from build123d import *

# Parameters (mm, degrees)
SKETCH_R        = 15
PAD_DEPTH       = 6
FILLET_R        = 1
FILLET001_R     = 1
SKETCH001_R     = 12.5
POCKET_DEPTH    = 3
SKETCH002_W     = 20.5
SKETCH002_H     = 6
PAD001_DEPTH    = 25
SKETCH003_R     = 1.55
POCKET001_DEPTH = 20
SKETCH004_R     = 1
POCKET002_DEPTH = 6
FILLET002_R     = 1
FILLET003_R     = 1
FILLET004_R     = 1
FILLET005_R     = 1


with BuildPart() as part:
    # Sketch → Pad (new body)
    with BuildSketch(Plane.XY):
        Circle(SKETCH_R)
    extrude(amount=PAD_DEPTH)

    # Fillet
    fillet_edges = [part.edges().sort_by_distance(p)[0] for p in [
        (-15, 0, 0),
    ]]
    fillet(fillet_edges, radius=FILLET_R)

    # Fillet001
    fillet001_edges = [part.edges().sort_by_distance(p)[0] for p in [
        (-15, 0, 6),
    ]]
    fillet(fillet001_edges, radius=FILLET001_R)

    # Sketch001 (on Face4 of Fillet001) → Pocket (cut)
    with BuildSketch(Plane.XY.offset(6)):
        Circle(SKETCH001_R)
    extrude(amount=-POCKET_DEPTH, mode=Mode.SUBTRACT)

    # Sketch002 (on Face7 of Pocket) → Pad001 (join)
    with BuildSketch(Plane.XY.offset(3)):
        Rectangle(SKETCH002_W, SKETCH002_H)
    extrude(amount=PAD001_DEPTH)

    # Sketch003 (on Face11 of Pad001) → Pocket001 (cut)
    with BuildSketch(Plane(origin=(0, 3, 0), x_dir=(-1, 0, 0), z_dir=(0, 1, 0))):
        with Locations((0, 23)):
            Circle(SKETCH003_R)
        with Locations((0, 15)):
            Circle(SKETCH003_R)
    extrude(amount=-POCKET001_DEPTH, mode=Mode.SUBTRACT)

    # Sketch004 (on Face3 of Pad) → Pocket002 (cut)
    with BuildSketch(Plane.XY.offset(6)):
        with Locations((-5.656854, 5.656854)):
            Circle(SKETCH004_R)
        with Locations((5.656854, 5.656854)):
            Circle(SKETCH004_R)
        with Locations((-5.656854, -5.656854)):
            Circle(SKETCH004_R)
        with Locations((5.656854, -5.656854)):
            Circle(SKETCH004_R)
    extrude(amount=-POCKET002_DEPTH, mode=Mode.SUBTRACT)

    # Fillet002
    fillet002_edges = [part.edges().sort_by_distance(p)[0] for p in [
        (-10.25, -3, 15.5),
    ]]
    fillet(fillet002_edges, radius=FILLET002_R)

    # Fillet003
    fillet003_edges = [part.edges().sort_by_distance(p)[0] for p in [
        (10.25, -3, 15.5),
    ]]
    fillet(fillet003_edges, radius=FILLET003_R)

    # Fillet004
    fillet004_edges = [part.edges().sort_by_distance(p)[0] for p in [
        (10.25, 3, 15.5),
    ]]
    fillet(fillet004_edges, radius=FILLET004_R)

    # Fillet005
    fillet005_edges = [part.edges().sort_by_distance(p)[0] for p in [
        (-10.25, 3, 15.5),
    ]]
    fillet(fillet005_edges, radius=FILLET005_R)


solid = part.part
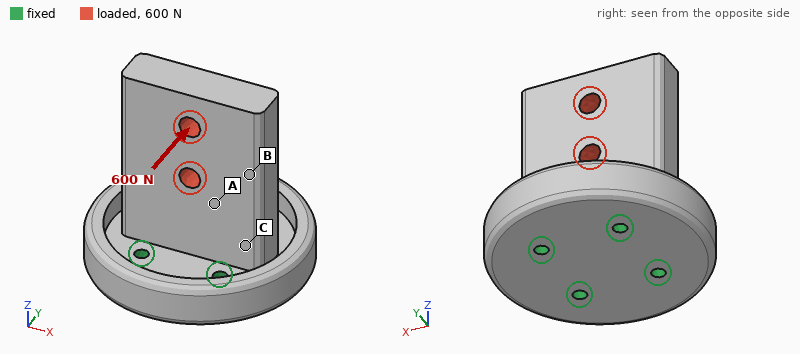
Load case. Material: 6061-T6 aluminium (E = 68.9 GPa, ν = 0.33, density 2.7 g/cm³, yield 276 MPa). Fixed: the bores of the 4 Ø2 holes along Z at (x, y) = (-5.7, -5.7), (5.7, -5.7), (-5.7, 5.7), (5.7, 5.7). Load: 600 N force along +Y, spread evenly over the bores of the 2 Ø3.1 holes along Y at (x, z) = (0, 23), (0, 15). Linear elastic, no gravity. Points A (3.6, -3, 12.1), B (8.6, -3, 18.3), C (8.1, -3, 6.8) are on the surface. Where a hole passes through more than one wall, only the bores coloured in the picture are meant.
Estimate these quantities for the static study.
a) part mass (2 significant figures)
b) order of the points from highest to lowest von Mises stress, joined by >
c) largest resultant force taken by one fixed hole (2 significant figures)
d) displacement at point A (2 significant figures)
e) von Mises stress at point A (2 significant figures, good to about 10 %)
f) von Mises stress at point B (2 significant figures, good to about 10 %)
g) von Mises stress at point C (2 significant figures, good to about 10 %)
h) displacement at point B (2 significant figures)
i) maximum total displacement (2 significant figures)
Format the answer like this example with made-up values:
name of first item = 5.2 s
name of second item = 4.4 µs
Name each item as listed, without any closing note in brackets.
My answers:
part mass = 15 g
order of the points from highest to lowest von Mises stress, joined by > = C > A > B
largest resultant force taken by one fixed hole = 550 N
displacement at point A = 29 µm
von Mises stress at point A = 37 MPa
von Mises stress at point B = 14 MPa
von Mises stress at point C = 62 MPa
displacement at point B = 53 µm
maximum total displacement = 99 µm
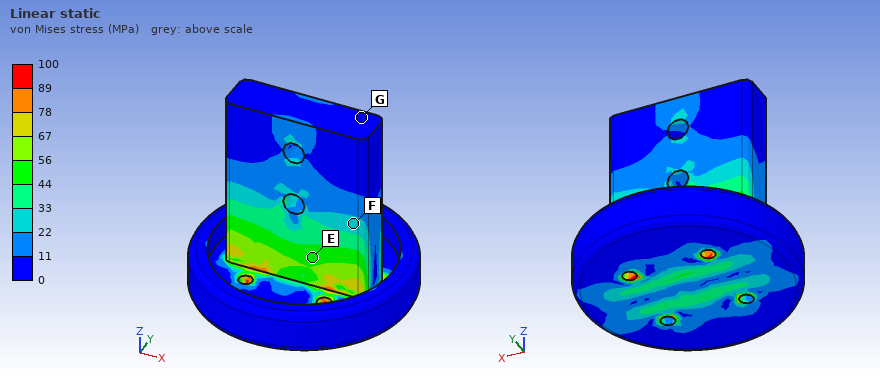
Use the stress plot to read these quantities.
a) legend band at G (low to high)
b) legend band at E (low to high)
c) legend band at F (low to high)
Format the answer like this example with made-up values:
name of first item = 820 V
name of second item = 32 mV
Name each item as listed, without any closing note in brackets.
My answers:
legend band at G = 0 to 11 MPa
legend band at E = 44 to 56 MPa
legend band at F = 22 to 33 MPa
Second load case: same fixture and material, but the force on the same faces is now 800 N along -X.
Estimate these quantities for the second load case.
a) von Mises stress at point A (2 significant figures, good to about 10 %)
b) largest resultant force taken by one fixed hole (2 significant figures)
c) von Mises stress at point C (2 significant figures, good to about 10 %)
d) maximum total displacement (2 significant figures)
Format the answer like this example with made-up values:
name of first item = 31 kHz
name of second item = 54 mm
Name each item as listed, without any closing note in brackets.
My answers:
von Mises stress at point A = 14 MPa
largest resultant force taken by one fixed hole = 560 N
von Mises stress at point C = 19 MPa
maximum total displacement = 34 µm
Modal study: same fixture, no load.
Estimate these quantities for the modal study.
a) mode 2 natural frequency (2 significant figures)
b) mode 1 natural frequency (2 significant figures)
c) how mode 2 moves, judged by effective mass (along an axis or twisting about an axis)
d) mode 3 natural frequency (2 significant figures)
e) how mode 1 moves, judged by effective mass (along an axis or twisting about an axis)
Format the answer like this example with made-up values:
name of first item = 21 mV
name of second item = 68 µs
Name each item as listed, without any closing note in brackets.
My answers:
mode 2 natural frequency = 11 kHz
mode 1 natural frequency = 6300 Hz
how mode 2 moves, judged by effective mass = along X
mode 3 natural frequency = 16 kHz
how mode 1 moves, judged by effective mass = along Y
